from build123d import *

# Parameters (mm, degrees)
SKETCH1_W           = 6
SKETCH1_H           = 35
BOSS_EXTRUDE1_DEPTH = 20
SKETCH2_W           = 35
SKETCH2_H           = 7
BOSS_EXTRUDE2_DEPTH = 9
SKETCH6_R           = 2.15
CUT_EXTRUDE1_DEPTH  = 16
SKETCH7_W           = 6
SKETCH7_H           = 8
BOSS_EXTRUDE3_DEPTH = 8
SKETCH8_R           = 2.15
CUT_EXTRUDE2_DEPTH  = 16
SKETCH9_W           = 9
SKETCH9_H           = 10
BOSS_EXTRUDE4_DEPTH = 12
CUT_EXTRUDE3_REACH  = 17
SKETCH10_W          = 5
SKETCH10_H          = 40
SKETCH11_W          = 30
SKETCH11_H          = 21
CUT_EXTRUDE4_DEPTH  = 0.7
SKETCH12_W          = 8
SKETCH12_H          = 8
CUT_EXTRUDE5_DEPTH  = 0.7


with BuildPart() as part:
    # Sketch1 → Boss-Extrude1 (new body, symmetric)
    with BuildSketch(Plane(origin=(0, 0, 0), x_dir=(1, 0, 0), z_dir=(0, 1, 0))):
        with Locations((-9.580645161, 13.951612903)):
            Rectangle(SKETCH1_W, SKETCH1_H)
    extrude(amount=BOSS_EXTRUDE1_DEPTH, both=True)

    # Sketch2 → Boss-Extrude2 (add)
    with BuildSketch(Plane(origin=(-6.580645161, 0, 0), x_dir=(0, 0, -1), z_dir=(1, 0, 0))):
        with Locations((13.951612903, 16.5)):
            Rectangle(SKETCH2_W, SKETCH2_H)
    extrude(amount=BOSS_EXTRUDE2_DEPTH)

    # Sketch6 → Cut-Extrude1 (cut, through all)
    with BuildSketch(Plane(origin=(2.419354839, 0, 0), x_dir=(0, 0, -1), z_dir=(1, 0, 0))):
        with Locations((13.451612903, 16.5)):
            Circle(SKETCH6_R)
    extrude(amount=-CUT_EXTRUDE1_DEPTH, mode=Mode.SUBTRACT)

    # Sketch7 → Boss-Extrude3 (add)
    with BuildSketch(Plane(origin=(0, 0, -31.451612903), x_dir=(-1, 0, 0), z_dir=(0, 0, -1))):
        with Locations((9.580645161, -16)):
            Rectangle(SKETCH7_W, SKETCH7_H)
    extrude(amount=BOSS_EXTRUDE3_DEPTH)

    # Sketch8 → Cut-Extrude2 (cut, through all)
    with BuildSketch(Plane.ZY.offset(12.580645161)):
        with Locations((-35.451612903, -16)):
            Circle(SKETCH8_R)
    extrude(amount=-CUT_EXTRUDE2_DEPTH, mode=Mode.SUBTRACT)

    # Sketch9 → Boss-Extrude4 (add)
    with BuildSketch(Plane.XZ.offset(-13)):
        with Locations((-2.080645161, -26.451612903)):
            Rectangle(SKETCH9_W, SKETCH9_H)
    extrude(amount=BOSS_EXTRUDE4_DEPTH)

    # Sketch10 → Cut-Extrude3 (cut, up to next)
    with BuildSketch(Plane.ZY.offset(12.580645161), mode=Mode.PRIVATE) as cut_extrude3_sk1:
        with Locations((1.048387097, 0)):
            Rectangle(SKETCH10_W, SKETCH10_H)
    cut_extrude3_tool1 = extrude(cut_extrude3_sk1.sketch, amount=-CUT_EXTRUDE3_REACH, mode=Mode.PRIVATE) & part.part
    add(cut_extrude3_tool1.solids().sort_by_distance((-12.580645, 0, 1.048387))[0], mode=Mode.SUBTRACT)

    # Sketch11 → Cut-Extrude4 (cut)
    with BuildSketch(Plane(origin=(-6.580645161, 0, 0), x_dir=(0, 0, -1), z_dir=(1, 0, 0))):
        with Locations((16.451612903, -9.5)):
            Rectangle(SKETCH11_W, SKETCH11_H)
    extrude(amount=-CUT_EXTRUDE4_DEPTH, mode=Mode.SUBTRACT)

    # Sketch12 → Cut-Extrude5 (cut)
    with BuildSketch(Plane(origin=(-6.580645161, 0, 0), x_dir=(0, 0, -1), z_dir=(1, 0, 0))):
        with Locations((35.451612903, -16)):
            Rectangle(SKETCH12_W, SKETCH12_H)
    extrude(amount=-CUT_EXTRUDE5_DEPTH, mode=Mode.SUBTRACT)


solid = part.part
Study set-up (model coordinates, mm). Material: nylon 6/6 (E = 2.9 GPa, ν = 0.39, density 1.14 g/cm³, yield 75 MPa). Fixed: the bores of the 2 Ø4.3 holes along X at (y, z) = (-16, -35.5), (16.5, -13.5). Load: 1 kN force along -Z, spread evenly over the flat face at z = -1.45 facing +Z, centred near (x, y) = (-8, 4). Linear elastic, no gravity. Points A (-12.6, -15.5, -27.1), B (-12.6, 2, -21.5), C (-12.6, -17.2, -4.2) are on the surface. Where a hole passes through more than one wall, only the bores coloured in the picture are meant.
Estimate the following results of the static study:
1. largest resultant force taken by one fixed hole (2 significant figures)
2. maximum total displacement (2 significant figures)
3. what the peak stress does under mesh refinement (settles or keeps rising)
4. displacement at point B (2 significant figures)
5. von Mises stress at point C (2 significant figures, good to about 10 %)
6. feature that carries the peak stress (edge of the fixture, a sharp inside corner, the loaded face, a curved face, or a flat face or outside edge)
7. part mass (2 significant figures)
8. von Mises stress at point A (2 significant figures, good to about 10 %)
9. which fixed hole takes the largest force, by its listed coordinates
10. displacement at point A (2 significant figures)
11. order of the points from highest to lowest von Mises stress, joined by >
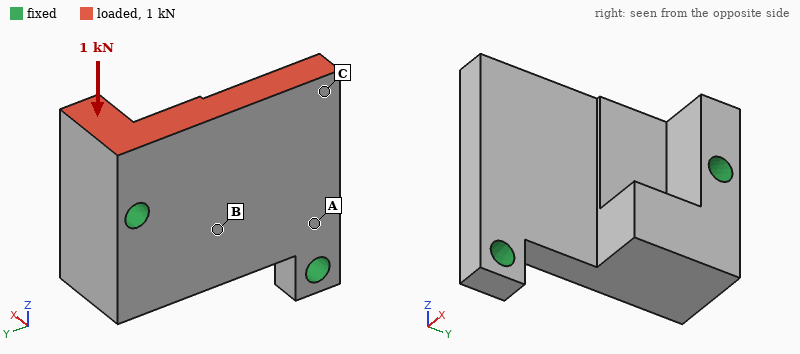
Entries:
630 N
72 µm
keeps rising
35 µm
3.5 MPa
edge of the fixture
11 g
8.2 MPa
(16.5, -13.5)
22 µm
A > C > B
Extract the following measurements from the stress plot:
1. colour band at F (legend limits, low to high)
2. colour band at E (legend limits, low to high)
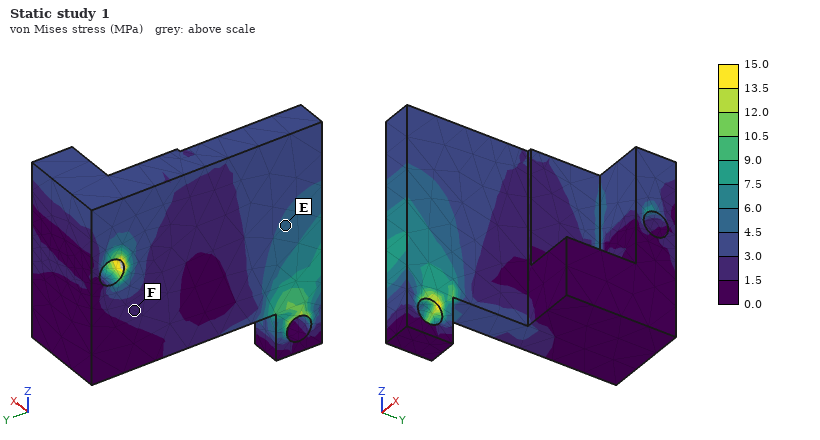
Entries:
1.5 to 3.0 MPa
4.5 to 6.0 MPa
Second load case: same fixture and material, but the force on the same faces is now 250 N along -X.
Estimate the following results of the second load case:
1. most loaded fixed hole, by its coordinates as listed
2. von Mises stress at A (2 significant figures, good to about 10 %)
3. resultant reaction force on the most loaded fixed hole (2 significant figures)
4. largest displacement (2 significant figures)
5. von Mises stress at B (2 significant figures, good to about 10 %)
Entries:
(16.5, -13.5)
8.3 MPa
220 N
0.60 mm
6.8 MPa
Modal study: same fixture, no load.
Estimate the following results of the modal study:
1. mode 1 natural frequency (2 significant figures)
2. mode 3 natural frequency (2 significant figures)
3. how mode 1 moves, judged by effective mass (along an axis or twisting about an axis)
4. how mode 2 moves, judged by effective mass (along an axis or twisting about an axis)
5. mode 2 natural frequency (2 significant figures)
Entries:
2300 Hz
6400 Hz
along X
along X
5200 Hz
